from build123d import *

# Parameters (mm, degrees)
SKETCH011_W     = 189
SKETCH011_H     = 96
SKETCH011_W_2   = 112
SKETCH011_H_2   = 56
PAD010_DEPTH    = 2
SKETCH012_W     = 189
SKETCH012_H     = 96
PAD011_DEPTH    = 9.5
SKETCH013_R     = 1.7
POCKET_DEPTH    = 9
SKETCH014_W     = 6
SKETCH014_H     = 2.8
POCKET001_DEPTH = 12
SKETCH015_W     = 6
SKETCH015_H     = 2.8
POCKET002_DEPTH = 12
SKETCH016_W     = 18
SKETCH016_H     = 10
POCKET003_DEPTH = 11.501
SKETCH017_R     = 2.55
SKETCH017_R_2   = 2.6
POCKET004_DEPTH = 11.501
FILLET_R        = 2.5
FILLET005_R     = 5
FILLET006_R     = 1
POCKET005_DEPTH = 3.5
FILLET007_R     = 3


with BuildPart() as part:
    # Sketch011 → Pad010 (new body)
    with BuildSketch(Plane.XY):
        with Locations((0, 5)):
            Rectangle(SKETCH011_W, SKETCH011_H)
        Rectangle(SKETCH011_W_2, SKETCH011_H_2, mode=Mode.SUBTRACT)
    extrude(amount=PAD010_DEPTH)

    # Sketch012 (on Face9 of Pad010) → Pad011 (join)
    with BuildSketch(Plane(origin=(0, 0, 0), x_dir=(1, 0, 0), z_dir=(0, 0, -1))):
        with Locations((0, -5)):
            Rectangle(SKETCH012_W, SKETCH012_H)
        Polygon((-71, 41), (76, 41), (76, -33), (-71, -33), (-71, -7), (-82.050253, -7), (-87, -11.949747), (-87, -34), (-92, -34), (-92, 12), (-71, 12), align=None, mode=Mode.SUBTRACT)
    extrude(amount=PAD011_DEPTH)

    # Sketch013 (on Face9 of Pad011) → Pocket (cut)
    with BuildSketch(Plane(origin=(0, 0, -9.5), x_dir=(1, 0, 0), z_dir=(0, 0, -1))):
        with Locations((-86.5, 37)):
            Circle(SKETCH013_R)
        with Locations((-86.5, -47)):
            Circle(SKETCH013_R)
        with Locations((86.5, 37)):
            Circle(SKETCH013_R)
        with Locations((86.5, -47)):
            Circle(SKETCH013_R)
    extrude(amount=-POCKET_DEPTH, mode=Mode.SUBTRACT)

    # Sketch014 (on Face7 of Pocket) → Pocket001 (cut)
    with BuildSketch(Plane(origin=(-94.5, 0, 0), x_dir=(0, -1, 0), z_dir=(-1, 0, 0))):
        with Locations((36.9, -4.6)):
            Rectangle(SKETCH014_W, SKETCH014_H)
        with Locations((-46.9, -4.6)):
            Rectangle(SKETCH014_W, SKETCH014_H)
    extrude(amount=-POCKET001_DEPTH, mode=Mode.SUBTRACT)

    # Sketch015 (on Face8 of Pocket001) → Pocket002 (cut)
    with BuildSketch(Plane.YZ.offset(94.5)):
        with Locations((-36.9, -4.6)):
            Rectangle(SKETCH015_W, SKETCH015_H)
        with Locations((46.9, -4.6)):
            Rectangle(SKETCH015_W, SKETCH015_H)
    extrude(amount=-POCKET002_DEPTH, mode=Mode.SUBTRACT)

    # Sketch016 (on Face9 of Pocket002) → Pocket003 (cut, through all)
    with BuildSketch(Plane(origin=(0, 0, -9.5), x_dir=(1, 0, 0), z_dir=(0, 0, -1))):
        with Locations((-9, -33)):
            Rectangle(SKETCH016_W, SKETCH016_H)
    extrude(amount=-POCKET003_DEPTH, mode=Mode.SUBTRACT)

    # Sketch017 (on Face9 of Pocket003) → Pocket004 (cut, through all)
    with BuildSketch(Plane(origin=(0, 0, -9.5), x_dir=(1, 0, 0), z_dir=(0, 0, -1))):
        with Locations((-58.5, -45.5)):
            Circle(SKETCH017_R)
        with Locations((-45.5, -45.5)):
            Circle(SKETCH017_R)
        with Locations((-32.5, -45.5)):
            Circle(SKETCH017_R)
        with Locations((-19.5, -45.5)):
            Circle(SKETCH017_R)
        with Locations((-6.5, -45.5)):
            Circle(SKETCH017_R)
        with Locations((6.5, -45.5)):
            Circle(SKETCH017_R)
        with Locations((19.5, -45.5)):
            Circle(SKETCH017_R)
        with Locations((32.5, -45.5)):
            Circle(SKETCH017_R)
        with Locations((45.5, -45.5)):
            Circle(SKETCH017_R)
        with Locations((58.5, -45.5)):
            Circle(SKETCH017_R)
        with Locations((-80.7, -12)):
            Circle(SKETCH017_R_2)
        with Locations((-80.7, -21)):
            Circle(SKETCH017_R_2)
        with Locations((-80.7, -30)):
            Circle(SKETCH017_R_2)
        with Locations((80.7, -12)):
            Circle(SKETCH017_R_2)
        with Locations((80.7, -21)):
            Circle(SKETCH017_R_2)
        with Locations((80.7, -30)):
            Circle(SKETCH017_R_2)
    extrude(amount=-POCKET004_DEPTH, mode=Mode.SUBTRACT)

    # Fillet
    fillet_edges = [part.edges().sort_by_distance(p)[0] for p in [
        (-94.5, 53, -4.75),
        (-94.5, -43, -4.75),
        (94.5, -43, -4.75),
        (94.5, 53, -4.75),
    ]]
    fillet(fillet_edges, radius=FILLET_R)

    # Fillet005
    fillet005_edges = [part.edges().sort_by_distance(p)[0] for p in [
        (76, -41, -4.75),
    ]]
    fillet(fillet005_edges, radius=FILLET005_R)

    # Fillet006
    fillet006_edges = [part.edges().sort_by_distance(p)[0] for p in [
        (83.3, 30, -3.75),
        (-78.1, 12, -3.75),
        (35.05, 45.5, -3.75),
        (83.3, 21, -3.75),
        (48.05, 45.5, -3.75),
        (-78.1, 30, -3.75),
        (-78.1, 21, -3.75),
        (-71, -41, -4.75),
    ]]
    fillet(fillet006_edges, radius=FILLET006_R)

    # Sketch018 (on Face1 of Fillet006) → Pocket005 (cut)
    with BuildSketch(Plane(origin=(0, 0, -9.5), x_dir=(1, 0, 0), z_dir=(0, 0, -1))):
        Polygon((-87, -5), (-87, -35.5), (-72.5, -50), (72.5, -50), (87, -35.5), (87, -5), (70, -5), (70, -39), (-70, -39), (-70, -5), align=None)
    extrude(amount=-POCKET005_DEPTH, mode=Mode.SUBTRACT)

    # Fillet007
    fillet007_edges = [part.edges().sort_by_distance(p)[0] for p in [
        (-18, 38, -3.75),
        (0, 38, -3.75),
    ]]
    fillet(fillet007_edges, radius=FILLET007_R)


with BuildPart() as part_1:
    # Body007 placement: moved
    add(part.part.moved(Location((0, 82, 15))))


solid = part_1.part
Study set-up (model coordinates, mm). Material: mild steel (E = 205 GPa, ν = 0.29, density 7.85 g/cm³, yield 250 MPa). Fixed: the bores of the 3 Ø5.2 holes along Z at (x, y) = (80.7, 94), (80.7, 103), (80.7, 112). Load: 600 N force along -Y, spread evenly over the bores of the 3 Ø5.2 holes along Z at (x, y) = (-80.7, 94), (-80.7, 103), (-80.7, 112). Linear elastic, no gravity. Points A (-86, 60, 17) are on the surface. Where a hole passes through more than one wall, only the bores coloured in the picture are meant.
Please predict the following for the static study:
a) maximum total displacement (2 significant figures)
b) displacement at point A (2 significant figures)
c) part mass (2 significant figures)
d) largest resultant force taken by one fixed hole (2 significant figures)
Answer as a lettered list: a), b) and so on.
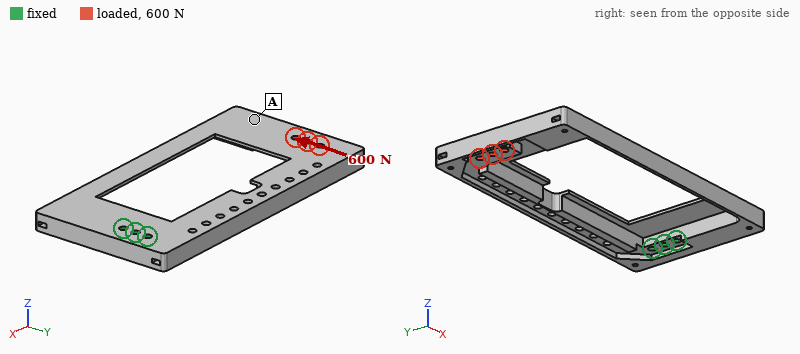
a) 0.26 mm
b) 0.19 mm
c) 580 g
d) 3.8 kN
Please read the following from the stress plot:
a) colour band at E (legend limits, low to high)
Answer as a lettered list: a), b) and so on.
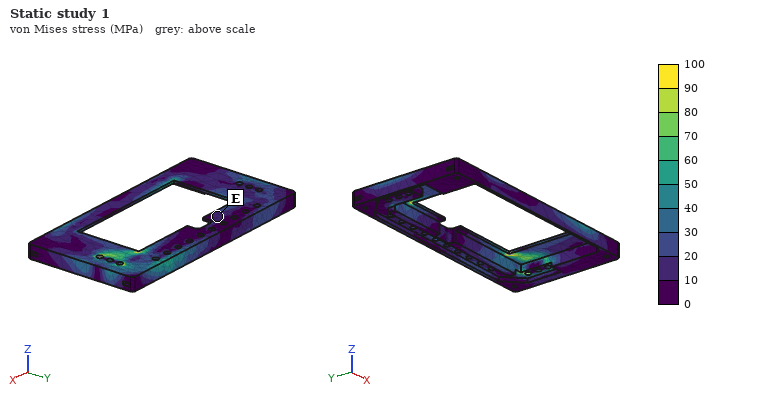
a) 10 to 20 MPa
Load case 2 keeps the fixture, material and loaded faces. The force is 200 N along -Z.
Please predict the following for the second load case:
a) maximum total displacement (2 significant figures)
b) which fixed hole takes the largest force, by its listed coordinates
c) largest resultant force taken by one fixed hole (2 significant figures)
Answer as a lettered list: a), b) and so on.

a) 0.90 mm
b) (80.7, 103)
c) 590 N
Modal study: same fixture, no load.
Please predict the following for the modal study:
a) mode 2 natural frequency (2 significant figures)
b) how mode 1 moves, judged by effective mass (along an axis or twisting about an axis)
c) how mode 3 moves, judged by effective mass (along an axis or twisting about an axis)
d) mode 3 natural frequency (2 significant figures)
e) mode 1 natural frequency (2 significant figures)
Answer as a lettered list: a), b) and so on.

a) 410 Hz
b) along Z
c) along Y
d) 610 Hz
e) 170 Hz
